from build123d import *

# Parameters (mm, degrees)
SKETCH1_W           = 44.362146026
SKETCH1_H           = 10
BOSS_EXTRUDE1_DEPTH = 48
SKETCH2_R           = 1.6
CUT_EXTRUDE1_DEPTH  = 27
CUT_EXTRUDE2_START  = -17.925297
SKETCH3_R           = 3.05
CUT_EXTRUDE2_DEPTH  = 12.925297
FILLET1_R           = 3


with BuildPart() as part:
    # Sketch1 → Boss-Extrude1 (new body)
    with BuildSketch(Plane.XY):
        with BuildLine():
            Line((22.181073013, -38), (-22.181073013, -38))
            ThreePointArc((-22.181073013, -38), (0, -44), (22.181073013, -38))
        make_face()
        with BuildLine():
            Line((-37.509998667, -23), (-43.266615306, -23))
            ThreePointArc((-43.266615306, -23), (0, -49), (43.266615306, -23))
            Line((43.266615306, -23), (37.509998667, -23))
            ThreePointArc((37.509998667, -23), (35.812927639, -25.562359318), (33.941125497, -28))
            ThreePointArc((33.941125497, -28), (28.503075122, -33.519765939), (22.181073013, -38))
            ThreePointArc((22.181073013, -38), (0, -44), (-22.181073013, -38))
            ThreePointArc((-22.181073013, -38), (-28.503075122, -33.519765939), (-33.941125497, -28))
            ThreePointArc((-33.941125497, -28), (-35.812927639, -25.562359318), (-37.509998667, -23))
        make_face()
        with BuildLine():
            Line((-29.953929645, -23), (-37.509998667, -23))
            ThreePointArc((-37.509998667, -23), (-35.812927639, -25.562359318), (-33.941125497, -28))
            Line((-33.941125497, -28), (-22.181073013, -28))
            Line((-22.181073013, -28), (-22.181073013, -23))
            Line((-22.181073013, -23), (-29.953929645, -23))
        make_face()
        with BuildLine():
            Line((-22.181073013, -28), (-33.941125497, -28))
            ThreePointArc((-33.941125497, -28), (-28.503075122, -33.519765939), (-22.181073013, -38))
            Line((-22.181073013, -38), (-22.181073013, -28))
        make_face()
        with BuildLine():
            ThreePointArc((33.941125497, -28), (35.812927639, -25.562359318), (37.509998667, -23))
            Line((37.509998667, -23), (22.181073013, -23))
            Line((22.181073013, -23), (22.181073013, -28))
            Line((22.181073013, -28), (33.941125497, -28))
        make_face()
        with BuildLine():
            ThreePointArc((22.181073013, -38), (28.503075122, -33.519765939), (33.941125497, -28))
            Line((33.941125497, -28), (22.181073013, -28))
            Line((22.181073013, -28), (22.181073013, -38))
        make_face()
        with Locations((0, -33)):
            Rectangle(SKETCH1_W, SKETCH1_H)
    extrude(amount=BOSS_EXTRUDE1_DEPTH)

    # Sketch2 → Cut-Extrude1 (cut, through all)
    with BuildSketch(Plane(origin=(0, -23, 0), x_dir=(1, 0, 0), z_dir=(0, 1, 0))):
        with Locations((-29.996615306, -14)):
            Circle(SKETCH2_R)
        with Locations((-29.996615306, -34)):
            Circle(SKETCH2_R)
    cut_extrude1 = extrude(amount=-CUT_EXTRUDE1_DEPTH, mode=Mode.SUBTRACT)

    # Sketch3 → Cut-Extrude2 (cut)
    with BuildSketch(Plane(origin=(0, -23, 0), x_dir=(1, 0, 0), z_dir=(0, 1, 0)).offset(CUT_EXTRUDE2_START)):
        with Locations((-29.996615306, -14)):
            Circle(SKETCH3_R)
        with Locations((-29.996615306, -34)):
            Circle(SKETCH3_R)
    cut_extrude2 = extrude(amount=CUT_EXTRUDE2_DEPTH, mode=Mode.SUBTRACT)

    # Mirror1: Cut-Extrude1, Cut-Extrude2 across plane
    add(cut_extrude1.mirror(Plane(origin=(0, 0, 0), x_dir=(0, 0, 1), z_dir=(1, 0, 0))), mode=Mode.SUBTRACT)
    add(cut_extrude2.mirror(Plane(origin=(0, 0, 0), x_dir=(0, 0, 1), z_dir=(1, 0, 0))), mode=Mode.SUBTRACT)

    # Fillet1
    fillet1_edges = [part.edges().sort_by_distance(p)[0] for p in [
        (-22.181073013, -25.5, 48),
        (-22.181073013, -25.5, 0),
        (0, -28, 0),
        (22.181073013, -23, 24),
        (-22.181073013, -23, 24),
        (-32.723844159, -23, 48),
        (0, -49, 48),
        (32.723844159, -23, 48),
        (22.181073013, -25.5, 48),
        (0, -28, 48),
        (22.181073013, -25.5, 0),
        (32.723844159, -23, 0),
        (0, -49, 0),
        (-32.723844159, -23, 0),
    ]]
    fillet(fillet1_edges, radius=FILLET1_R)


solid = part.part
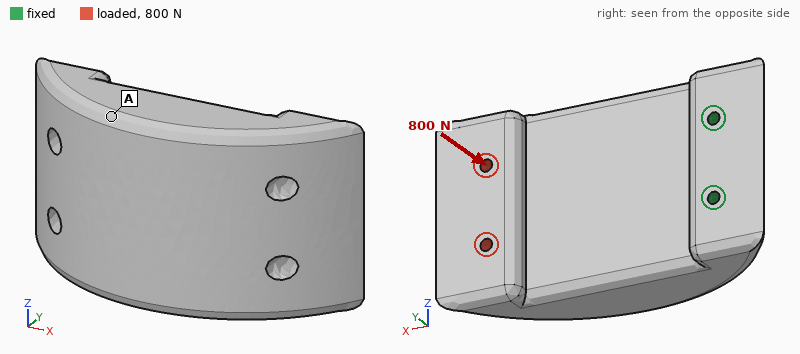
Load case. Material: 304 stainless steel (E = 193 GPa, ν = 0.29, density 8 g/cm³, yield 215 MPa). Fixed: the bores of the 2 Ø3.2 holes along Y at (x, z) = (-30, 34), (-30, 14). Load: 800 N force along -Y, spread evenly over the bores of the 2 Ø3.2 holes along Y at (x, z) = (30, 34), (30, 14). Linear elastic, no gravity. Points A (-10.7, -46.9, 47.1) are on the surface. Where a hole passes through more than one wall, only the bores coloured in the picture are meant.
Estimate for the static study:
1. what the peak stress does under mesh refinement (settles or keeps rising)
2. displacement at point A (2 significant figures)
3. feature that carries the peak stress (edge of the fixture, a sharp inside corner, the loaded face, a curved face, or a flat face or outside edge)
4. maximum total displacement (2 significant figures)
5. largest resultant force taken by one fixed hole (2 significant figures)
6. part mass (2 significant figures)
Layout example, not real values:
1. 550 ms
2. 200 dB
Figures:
1. keeps rising
2. 0.055 mm
3. edge of the fixture
4. 0.15 mm
5. 450 N
6. 510 g
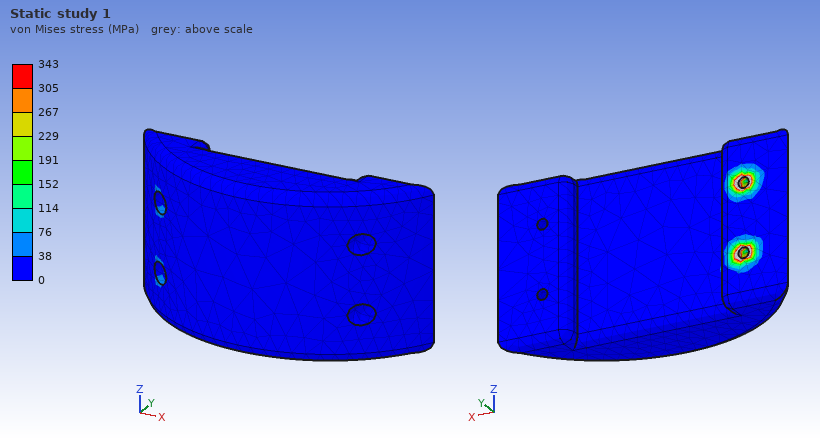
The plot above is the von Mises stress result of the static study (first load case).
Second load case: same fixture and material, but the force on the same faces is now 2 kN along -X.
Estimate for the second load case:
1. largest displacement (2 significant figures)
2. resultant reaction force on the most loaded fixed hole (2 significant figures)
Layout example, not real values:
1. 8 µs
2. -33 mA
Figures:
1. 17 µm
2. 1.0 kN
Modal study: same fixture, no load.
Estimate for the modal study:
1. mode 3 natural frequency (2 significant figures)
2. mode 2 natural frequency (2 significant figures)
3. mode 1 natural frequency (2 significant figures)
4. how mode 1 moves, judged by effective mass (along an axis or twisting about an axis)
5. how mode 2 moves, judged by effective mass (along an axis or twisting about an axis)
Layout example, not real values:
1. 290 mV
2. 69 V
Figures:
1. 5100 Hz
2. 2500 Hz
3. 910 Hz
4. along Y
5. along Z
